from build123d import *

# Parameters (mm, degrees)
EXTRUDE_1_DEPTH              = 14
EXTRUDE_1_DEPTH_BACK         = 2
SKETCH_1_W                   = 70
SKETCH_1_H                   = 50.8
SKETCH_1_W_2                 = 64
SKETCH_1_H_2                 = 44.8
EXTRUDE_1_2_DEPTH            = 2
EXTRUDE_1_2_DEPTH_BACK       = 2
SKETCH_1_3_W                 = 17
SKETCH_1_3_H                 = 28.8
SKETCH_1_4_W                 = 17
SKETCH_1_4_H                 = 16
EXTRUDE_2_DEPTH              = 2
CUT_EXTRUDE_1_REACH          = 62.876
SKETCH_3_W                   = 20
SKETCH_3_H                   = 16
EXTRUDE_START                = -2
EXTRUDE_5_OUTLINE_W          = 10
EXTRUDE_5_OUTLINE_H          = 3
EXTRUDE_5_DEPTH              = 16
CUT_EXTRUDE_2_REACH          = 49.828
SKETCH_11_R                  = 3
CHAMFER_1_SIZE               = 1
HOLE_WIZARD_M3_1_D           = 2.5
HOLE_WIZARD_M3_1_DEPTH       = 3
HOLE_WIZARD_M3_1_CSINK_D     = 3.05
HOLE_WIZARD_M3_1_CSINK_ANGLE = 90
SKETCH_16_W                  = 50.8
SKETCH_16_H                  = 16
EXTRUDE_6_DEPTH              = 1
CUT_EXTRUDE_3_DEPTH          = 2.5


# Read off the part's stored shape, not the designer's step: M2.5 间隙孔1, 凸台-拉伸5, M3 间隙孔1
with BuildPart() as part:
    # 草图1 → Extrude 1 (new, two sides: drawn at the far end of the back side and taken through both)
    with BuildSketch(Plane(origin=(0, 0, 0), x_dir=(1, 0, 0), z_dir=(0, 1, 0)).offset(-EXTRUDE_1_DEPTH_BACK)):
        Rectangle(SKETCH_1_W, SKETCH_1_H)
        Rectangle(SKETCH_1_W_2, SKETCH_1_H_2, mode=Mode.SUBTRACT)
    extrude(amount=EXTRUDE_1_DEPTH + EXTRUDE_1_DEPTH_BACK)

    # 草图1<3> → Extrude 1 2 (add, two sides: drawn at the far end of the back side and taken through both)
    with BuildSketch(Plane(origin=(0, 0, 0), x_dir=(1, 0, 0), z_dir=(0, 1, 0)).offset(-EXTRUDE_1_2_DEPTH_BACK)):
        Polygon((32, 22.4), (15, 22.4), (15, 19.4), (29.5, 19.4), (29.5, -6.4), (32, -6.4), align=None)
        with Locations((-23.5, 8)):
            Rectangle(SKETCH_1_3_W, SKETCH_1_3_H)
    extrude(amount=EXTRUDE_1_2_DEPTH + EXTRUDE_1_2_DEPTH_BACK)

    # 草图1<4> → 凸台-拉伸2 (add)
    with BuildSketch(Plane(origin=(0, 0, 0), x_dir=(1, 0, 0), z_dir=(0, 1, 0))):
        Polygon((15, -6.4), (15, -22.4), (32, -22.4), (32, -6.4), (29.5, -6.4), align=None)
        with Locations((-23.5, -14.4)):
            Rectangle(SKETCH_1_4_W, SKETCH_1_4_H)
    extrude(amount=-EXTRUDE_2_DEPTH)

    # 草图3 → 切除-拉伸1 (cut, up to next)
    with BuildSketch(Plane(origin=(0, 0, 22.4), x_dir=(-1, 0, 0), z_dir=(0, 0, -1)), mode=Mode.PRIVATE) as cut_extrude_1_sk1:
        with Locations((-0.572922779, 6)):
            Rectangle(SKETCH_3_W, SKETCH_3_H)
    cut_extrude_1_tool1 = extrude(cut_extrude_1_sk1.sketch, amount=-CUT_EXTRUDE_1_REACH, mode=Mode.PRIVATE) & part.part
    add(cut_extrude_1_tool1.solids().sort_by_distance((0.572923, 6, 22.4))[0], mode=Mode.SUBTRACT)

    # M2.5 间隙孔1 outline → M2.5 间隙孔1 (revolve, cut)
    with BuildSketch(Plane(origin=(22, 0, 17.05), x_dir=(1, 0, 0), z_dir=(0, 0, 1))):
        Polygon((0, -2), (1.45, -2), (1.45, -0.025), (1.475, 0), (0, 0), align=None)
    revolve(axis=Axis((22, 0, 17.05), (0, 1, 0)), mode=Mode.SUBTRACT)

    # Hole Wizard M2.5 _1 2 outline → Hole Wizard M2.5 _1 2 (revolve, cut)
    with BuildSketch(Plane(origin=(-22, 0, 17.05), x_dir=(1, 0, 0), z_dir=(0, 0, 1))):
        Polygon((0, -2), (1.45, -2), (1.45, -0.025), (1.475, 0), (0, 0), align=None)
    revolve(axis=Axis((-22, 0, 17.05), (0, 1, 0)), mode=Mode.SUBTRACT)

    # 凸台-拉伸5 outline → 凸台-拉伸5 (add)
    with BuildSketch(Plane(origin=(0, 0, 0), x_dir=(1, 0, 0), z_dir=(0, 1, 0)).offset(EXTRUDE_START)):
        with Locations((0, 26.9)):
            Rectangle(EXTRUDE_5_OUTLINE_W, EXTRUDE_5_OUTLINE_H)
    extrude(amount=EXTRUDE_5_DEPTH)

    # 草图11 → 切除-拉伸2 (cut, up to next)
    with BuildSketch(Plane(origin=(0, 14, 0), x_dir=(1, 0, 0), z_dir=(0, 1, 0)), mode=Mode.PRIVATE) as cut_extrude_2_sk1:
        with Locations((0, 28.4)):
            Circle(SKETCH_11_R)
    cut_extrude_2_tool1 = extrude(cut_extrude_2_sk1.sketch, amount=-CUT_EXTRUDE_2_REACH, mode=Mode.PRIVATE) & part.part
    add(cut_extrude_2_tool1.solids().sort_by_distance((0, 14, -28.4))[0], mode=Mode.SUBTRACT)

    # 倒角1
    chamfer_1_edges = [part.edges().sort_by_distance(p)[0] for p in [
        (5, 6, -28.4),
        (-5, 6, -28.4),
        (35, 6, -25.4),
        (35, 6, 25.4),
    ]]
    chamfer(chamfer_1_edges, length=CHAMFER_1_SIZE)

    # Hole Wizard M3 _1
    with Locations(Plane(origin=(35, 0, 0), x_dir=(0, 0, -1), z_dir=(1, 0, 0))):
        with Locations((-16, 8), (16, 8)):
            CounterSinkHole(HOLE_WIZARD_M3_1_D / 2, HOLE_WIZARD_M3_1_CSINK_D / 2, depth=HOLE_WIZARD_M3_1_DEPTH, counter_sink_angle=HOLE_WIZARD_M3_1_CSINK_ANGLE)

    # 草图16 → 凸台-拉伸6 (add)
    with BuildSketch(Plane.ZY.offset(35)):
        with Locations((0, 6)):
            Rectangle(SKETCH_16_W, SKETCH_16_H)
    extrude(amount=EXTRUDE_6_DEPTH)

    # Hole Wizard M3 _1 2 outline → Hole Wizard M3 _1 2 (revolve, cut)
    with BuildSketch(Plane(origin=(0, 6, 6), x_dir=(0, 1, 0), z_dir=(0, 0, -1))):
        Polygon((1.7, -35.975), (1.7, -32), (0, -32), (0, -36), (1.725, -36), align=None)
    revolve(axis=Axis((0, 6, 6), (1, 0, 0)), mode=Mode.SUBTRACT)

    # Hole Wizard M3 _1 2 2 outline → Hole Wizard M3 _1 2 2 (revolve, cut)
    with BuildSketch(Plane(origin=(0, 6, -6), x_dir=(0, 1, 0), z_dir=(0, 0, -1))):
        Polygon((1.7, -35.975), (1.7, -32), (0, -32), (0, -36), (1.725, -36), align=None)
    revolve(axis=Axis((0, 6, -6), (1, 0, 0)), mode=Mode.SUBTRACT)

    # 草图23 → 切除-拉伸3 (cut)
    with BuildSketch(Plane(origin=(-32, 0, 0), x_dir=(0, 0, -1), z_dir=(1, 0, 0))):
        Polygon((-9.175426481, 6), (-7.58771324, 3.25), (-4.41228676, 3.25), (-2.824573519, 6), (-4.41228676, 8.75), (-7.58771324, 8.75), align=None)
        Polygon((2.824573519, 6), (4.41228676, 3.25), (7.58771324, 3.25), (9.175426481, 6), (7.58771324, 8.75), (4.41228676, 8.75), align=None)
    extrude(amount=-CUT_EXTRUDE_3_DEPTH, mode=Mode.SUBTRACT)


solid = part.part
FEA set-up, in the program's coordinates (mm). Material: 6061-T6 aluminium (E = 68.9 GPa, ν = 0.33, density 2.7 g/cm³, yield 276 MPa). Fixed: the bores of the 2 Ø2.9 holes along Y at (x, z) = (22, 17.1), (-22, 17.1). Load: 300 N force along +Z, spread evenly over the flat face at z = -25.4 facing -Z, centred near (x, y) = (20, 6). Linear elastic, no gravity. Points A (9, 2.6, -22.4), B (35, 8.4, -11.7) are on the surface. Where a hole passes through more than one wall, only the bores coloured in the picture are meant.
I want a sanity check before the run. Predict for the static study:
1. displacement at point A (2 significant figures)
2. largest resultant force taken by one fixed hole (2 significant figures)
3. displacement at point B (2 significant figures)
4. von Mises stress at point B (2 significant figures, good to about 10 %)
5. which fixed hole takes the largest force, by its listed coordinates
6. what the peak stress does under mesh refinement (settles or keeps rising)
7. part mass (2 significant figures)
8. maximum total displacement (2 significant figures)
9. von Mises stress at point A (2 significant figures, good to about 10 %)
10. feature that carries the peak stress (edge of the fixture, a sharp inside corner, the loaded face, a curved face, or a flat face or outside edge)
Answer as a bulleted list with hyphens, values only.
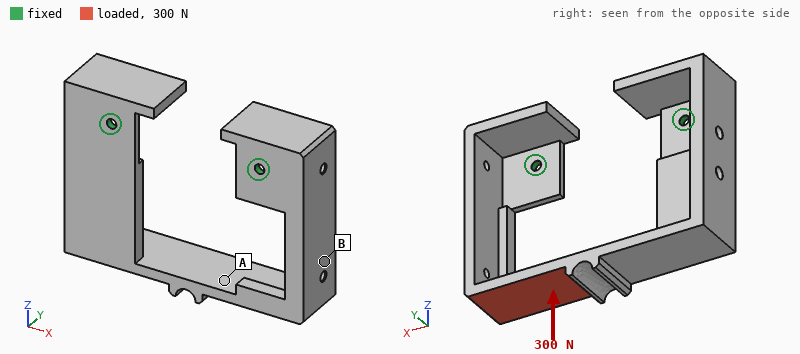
- 0.19 mm
- 230 N
- 0.17 mm
- 12 MPa
- (22, 17.1)
- keeps rising
- 39 g
- 0.25 mm
- 37 MPa
- edge of the fixture
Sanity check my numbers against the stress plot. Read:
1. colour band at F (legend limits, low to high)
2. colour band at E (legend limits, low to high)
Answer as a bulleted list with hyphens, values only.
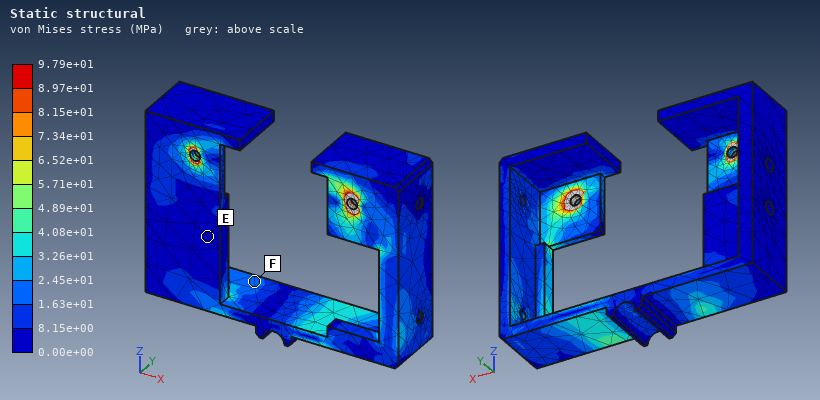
- 1.63e+01 to 2.45e+01 MPa
- 0.00e+00 to 8.15e+00 MPa
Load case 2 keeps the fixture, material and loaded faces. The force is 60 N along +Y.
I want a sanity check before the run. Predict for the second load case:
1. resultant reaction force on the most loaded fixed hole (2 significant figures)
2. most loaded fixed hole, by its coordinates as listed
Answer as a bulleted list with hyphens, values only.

- 38 N
- (22, 17.1)
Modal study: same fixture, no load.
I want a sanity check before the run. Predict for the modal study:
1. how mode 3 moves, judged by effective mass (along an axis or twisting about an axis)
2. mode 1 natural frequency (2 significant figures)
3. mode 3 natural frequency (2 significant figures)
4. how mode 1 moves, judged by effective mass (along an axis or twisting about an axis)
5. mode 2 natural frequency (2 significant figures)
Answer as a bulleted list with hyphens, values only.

- along X
- 670 Hz
- 1600 Hz
- along Y
- 1100 Hz
